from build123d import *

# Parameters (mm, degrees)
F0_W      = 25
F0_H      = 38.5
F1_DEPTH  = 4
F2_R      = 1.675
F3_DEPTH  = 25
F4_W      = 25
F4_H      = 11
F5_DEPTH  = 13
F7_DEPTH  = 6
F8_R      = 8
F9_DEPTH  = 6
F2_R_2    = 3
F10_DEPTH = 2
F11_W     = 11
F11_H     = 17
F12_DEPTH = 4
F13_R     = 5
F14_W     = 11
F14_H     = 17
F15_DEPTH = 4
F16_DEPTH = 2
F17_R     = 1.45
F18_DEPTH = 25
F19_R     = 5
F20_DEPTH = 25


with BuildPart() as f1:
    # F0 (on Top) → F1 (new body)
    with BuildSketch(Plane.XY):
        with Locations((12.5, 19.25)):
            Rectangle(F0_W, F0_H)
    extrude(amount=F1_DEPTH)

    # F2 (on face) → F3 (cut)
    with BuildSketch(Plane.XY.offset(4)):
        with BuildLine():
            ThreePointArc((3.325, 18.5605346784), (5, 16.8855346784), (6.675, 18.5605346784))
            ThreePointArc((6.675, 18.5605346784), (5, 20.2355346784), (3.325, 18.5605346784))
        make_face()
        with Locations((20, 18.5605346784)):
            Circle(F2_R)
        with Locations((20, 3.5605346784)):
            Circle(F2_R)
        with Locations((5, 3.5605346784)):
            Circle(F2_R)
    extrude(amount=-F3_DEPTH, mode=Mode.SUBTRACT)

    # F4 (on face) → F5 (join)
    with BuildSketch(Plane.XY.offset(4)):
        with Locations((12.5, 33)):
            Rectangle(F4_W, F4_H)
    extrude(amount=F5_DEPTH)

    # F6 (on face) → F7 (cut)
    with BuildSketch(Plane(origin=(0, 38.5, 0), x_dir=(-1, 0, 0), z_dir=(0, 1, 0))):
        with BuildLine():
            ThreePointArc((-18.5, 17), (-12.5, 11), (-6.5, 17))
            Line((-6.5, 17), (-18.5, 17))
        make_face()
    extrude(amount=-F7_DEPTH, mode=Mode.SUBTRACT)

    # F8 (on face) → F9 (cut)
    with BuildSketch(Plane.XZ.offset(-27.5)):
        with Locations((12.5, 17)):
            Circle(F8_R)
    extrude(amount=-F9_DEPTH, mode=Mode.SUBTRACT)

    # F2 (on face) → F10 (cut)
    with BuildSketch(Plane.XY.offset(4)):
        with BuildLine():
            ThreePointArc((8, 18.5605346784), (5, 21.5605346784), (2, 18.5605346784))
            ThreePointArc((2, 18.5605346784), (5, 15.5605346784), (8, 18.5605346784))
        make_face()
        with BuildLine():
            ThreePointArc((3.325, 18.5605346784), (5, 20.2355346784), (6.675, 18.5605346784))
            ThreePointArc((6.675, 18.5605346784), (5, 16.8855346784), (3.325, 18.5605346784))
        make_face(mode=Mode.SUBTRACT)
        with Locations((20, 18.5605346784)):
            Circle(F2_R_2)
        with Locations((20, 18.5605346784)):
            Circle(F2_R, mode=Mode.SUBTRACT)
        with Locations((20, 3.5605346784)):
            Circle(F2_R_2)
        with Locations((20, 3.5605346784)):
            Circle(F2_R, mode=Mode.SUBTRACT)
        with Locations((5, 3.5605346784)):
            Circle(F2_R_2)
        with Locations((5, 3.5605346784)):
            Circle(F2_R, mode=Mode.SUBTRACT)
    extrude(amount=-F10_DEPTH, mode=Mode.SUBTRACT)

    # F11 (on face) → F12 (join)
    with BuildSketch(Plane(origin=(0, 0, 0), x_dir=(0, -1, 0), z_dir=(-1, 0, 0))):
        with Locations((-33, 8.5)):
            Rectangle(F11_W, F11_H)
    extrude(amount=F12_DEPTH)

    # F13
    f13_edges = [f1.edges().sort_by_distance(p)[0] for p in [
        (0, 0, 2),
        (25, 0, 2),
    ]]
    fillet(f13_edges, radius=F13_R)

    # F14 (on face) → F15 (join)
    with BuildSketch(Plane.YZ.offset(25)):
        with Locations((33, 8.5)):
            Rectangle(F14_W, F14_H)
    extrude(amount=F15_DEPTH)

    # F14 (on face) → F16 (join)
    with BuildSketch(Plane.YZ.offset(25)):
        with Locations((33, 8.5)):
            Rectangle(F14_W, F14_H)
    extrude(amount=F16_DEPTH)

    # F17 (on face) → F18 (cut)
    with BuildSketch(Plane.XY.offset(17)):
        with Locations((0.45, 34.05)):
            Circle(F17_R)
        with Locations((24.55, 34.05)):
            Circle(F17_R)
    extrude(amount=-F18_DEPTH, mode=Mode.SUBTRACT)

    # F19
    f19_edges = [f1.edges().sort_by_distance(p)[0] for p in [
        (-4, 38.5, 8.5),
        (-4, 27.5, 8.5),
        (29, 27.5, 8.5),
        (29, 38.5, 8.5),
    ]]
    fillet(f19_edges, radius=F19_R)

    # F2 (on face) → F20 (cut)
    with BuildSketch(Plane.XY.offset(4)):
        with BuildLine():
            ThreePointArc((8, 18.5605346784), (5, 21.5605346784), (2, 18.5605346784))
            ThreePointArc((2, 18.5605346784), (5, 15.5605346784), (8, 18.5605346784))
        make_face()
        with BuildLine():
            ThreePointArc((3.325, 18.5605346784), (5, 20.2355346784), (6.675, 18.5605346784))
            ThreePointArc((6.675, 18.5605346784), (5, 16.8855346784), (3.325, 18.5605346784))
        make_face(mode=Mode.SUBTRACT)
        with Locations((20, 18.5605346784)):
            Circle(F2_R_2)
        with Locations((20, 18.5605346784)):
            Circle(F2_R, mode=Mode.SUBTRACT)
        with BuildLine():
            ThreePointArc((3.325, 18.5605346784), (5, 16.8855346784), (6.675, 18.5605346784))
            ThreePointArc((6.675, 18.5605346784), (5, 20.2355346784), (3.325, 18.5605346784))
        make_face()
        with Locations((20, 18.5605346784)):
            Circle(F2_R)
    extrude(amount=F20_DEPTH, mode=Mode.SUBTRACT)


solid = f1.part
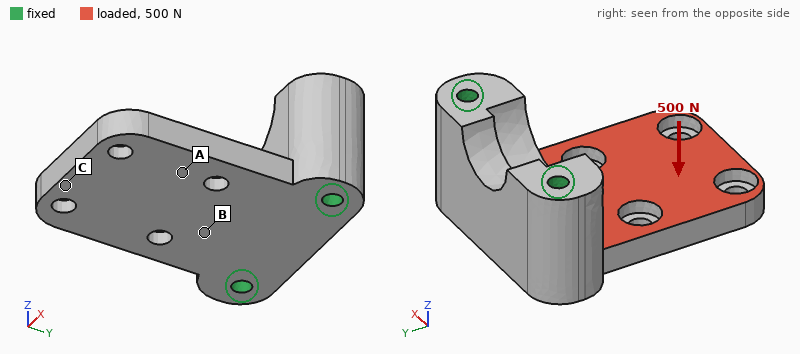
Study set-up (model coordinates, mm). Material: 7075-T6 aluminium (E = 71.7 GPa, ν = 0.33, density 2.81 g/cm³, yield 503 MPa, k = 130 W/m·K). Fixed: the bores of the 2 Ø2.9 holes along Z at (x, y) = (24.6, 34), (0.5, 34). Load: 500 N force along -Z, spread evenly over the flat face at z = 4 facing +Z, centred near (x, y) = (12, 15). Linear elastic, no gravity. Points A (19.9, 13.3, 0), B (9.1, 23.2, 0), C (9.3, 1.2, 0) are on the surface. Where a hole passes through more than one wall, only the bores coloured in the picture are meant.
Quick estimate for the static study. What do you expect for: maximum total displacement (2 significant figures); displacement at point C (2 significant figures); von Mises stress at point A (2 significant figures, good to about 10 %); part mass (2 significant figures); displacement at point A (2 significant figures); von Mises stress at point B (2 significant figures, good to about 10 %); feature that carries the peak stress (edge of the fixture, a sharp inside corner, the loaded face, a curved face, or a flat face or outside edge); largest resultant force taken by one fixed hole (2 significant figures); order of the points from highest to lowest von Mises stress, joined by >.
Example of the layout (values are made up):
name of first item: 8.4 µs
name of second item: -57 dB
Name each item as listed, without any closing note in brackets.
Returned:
maximum total displacement: 0.19 mm
displacement at point C: 0.18 mm
von Mises stress at point A: 19 MPa
part mass: 20 g
displacement at point A: 0.081 mm
von Mises stress at point B: 65 MPa
feature that carries the peak stress: the loaded face
largest resultant force taken by one fixed hole: 250 N
order of the points from highest to lowest von Mises stress, joined by >: B > A > C
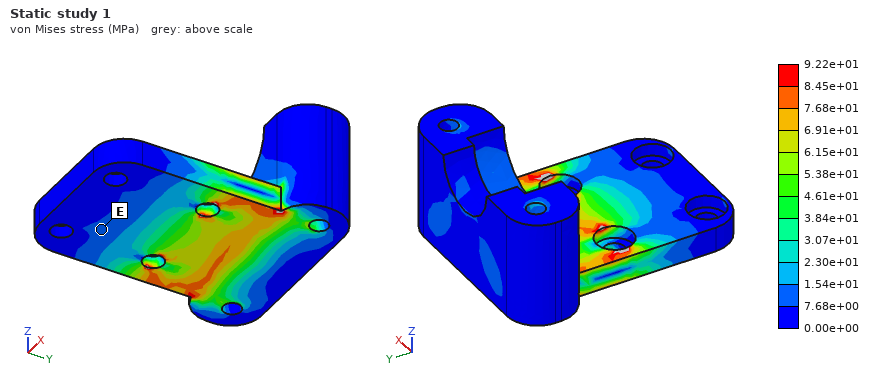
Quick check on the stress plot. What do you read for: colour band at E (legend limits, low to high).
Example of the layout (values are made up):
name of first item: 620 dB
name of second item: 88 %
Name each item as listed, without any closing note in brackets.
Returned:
colour band at E: 7.68e+00 to 1.54e+01 MPa
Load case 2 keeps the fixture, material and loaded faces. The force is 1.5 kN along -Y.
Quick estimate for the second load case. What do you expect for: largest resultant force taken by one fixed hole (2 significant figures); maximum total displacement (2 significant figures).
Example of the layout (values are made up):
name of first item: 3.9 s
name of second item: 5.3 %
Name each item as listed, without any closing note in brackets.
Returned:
largest resultant force taken by one fixed hole: 780 N
maximum total displacement: 0.11 mm
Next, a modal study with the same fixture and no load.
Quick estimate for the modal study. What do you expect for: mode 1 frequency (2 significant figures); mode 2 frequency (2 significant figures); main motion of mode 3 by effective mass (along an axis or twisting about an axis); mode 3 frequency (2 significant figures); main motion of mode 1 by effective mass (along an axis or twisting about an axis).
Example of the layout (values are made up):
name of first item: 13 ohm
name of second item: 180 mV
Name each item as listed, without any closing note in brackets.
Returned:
mode 1 frequency: 3900 Hz
mode 2 frequency: 10 kHz
main motion of mode 3 by effective mass: along X
mode 3 frequency: 16 kHz
main motion of mode 1 by effective mass: along Z
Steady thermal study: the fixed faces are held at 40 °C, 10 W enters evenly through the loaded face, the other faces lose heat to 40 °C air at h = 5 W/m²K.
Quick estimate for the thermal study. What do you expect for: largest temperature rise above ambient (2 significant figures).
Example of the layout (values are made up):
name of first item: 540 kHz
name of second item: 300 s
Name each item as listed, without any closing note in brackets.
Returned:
largest temperature rise above ambient: 15 K
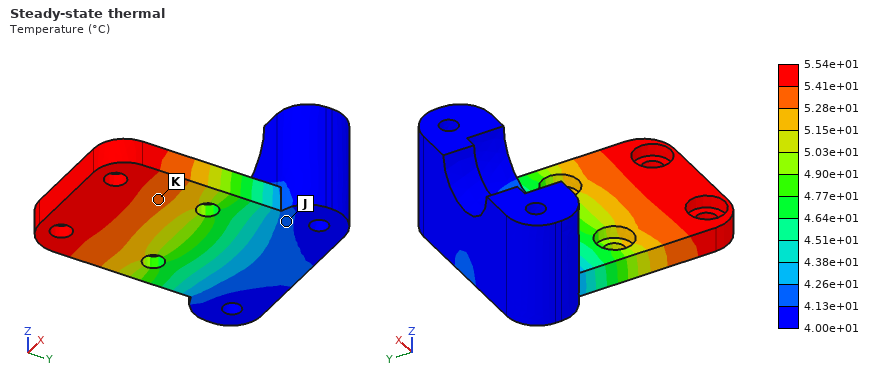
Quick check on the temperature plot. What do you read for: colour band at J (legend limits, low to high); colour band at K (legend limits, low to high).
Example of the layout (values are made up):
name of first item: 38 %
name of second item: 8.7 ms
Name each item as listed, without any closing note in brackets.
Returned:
colour band at J: 4.13e+01 to 4.26e+01 °C
colour band at K: 5.28e+01 to 5.41e+01 °C
